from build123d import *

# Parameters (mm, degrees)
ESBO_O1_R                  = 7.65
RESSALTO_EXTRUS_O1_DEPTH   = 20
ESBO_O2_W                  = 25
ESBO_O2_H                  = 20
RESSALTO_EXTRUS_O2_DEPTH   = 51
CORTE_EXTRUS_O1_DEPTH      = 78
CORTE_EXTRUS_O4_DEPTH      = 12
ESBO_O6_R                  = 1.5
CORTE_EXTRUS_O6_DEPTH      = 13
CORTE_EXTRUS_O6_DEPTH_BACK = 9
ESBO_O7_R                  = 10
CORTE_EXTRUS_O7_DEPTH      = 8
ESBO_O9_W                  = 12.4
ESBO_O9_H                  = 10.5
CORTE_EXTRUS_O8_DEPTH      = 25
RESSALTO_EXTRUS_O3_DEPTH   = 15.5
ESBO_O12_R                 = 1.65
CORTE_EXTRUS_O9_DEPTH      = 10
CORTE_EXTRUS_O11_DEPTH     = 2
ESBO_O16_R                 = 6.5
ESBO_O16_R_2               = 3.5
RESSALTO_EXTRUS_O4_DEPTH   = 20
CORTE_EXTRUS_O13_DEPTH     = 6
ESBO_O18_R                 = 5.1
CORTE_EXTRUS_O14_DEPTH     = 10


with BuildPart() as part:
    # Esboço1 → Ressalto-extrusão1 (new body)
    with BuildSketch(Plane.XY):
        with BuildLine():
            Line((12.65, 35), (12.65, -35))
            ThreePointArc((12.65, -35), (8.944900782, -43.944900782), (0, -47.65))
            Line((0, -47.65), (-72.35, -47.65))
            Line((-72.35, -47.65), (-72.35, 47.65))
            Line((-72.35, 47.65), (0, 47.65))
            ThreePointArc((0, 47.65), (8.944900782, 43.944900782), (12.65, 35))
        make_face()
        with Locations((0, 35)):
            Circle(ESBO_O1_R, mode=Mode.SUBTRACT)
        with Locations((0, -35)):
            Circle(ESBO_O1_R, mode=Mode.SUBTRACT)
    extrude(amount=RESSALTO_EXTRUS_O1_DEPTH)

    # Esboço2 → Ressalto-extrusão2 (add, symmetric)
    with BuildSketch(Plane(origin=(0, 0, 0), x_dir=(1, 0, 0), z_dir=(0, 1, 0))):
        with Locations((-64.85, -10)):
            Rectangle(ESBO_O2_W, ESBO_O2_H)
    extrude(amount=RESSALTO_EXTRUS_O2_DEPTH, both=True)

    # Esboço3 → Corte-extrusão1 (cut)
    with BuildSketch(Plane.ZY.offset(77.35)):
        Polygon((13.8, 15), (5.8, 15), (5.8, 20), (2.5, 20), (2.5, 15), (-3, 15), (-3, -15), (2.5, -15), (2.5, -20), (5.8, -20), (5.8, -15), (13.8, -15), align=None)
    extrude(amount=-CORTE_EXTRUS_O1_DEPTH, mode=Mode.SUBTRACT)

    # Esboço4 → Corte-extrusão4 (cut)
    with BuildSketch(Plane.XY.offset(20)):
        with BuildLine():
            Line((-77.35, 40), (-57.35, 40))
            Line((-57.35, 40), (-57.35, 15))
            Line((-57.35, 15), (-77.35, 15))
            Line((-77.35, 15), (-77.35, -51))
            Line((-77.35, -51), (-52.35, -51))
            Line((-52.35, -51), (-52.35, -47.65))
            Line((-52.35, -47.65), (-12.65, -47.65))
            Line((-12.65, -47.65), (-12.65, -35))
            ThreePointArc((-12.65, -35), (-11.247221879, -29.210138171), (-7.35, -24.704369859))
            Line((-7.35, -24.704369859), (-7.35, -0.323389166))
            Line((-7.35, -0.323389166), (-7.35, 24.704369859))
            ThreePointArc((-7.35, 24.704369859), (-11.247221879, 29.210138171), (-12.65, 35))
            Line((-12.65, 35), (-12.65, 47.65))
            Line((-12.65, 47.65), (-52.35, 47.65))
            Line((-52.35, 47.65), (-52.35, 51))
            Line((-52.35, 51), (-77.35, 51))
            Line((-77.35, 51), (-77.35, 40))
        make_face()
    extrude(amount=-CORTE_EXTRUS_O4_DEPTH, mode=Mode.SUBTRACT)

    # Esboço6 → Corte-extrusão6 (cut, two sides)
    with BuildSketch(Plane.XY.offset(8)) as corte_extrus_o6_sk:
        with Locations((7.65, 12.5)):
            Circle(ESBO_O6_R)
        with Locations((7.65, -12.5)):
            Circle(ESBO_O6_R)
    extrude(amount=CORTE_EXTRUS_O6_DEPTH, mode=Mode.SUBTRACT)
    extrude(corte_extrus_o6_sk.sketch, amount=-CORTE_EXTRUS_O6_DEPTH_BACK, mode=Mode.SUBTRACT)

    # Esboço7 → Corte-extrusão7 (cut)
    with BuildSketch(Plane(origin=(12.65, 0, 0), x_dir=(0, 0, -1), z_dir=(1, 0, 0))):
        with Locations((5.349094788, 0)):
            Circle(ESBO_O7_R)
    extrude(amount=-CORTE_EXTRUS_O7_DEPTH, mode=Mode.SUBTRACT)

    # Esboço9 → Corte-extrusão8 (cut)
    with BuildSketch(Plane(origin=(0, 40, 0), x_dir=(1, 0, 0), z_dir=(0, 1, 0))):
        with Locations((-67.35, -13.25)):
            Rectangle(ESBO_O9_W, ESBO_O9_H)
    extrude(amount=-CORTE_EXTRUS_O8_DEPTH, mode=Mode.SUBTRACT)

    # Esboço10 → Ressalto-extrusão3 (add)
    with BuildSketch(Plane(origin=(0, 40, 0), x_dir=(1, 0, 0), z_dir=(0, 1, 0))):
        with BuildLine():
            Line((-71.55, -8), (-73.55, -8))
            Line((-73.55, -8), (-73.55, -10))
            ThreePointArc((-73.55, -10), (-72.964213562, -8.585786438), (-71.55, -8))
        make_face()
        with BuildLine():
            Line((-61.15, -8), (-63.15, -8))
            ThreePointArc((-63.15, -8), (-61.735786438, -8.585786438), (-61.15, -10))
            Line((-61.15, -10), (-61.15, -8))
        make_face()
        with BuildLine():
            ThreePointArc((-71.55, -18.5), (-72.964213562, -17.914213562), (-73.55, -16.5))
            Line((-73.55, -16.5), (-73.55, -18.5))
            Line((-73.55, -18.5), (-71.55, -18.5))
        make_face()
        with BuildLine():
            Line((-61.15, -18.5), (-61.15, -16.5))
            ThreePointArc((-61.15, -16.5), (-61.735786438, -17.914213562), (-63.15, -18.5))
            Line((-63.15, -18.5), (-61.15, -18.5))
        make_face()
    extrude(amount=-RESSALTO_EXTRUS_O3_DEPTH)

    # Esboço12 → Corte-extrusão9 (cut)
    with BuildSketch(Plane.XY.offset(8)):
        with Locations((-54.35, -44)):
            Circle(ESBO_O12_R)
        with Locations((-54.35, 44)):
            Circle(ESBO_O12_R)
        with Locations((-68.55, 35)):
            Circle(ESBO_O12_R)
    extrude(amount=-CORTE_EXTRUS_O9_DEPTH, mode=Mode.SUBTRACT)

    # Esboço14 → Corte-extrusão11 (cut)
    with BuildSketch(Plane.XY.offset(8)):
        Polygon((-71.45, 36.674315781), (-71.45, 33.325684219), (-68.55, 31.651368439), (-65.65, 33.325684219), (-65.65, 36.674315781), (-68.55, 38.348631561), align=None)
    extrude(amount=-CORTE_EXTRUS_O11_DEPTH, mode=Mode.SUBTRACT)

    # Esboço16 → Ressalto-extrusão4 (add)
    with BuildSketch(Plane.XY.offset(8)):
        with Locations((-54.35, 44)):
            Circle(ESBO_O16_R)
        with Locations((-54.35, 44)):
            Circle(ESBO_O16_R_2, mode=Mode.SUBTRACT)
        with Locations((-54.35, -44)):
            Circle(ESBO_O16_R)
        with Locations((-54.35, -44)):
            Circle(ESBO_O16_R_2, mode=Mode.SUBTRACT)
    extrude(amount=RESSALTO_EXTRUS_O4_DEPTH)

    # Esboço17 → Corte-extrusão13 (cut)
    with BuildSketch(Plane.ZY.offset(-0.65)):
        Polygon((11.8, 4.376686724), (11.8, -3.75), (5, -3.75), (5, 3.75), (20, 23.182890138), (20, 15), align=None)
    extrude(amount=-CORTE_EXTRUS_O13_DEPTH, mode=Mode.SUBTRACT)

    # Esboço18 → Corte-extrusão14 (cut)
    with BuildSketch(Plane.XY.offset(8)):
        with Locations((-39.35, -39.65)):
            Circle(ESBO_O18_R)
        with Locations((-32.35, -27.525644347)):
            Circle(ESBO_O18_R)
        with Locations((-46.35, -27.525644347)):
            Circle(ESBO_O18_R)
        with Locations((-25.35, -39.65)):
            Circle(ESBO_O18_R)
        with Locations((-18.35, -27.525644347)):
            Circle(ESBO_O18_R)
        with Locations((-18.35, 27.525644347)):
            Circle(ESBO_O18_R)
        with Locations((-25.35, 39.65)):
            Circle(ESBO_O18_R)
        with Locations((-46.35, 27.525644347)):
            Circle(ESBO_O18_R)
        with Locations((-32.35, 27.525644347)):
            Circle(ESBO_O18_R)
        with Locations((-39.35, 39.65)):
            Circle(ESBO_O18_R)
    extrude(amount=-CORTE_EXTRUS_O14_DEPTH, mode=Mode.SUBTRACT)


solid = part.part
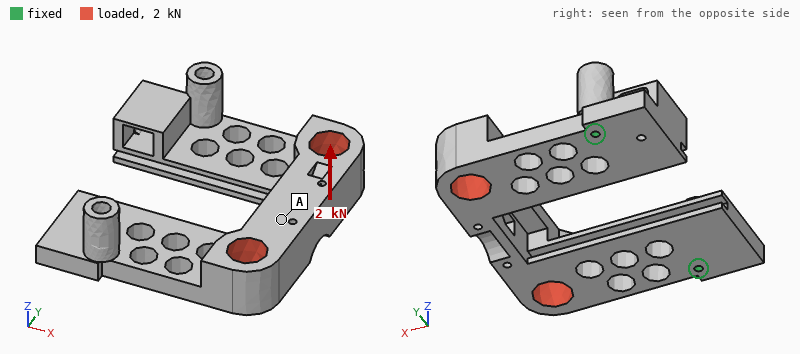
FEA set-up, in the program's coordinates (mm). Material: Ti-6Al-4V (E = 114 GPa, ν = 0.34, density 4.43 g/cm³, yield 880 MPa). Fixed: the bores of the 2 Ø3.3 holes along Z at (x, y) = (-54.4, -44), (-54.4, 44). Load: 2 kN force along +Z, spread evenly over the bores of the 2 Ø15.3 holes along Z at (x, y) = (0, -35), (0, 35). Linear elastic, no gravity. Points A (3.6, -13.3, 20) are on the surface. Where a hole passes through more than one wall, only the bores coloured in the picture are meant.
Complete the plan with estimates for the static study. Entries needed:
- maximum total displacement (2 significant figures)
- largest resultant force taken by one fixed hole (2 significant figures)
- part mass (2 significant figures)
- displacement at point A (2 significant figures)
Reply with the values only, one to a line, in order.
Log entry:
1.1 mm
1.0 kN
280 g
0.93 mm
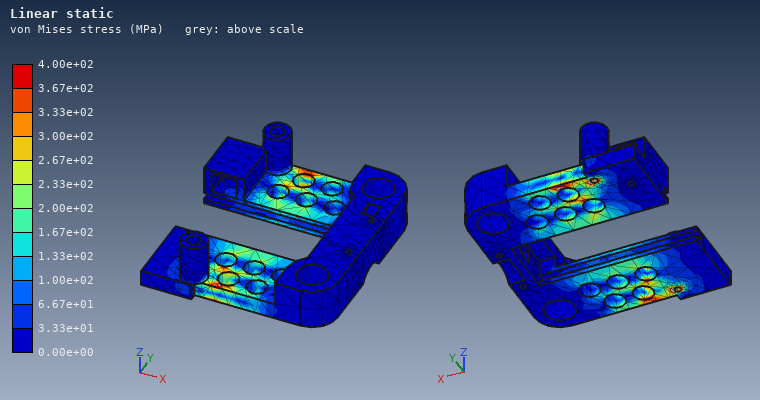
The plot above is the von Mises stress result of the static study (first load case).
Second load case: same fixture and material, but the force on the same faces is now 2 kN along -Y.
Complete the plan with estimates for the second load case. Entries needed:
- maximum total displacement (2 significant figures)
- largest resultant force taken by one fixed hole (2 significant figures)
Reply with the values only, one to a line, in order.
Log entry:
61 µm
1.5 kN
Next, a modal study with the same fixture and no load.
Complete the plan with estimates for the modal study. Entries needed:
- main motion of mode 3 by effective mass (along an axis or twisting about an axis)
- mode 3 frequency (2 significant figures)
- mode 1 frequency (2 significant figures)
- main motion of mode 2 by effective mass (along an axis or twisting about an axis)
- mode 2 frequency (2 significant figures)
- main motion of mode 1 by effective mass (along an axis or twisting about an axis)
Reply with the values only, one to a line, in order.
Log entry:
along Y
2500 Hz
640 Hz
twisting about X
1800 Hz
along Z
